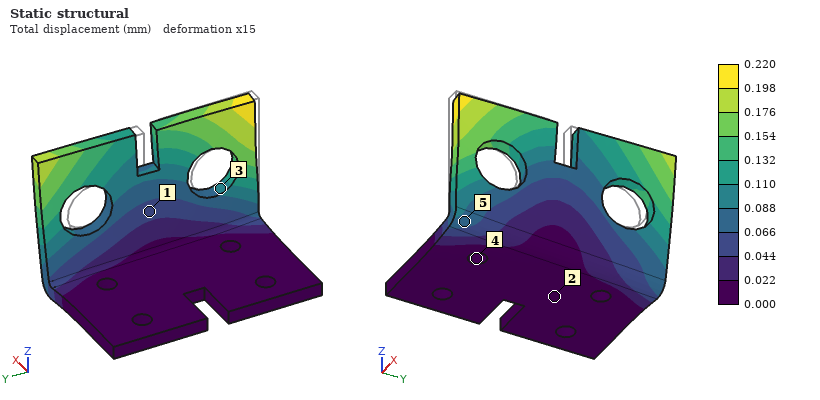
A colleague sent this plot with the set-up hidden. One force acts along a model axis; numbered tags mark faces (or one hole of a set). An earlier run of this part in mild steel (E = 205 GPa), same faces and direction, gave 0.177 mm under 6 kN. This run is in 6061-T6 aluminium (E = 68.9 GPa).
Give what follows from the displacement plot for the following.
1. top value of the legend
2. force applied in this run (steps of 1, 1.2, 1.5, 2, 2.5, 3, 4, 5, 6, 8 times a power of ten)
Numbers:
0.220 mm
2.5 kN
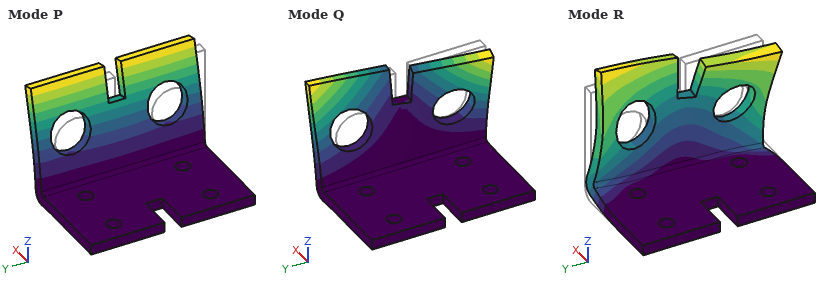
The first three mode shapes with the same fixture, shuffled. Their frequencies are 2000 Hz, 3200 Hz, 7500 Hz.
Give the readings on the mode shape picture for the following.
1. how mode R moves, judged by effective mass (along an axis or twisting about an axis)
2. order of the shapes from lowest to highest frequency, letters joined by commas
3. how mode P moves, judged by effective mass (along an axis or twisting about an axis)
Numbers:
along Y
P, Q, R
along X
